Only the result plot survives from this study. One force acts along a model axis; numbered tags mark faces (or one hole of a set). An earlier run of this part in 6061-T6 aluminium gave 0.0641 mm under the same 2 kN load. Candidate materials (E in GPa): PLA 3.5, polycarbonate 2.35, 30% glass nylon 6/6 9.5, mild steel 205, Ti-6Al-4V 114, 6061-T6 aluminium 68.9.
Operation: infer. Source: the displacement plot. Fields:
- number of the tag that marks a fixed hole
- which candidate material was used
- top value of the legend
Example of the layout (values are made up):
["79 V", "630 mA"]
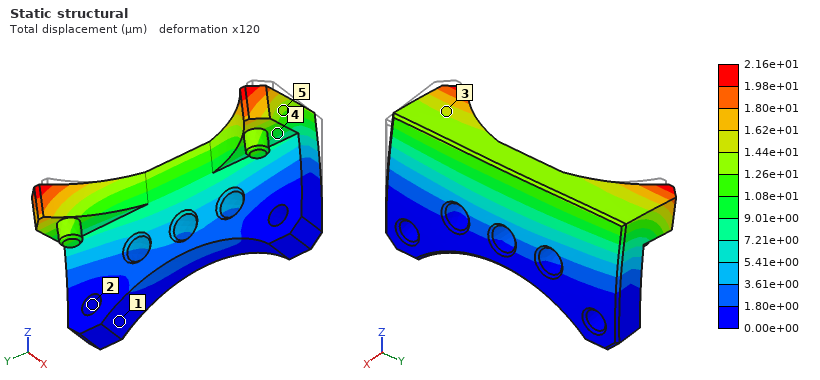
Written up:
["2", "mild steel", "2.16e+01 µm"]
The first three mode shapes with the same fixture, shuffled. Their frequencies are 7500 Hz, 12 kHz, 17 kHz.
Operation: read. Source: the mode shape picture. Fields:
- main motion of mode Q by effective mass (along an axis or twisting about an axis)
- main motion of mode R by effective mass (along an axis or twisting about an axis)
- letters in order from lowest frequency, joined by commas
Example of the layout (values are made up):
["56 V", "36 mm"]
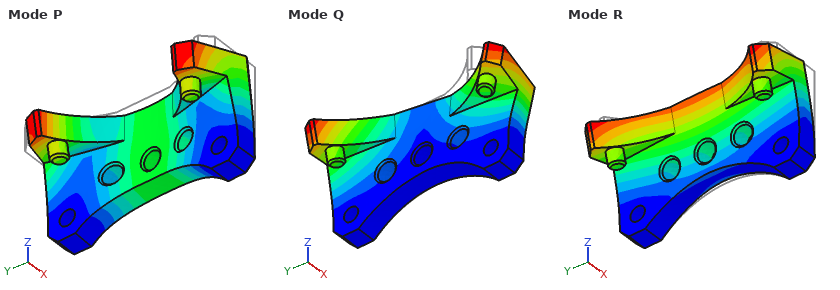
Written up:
["twisting about Z", "along X", "R, Q, P"]
